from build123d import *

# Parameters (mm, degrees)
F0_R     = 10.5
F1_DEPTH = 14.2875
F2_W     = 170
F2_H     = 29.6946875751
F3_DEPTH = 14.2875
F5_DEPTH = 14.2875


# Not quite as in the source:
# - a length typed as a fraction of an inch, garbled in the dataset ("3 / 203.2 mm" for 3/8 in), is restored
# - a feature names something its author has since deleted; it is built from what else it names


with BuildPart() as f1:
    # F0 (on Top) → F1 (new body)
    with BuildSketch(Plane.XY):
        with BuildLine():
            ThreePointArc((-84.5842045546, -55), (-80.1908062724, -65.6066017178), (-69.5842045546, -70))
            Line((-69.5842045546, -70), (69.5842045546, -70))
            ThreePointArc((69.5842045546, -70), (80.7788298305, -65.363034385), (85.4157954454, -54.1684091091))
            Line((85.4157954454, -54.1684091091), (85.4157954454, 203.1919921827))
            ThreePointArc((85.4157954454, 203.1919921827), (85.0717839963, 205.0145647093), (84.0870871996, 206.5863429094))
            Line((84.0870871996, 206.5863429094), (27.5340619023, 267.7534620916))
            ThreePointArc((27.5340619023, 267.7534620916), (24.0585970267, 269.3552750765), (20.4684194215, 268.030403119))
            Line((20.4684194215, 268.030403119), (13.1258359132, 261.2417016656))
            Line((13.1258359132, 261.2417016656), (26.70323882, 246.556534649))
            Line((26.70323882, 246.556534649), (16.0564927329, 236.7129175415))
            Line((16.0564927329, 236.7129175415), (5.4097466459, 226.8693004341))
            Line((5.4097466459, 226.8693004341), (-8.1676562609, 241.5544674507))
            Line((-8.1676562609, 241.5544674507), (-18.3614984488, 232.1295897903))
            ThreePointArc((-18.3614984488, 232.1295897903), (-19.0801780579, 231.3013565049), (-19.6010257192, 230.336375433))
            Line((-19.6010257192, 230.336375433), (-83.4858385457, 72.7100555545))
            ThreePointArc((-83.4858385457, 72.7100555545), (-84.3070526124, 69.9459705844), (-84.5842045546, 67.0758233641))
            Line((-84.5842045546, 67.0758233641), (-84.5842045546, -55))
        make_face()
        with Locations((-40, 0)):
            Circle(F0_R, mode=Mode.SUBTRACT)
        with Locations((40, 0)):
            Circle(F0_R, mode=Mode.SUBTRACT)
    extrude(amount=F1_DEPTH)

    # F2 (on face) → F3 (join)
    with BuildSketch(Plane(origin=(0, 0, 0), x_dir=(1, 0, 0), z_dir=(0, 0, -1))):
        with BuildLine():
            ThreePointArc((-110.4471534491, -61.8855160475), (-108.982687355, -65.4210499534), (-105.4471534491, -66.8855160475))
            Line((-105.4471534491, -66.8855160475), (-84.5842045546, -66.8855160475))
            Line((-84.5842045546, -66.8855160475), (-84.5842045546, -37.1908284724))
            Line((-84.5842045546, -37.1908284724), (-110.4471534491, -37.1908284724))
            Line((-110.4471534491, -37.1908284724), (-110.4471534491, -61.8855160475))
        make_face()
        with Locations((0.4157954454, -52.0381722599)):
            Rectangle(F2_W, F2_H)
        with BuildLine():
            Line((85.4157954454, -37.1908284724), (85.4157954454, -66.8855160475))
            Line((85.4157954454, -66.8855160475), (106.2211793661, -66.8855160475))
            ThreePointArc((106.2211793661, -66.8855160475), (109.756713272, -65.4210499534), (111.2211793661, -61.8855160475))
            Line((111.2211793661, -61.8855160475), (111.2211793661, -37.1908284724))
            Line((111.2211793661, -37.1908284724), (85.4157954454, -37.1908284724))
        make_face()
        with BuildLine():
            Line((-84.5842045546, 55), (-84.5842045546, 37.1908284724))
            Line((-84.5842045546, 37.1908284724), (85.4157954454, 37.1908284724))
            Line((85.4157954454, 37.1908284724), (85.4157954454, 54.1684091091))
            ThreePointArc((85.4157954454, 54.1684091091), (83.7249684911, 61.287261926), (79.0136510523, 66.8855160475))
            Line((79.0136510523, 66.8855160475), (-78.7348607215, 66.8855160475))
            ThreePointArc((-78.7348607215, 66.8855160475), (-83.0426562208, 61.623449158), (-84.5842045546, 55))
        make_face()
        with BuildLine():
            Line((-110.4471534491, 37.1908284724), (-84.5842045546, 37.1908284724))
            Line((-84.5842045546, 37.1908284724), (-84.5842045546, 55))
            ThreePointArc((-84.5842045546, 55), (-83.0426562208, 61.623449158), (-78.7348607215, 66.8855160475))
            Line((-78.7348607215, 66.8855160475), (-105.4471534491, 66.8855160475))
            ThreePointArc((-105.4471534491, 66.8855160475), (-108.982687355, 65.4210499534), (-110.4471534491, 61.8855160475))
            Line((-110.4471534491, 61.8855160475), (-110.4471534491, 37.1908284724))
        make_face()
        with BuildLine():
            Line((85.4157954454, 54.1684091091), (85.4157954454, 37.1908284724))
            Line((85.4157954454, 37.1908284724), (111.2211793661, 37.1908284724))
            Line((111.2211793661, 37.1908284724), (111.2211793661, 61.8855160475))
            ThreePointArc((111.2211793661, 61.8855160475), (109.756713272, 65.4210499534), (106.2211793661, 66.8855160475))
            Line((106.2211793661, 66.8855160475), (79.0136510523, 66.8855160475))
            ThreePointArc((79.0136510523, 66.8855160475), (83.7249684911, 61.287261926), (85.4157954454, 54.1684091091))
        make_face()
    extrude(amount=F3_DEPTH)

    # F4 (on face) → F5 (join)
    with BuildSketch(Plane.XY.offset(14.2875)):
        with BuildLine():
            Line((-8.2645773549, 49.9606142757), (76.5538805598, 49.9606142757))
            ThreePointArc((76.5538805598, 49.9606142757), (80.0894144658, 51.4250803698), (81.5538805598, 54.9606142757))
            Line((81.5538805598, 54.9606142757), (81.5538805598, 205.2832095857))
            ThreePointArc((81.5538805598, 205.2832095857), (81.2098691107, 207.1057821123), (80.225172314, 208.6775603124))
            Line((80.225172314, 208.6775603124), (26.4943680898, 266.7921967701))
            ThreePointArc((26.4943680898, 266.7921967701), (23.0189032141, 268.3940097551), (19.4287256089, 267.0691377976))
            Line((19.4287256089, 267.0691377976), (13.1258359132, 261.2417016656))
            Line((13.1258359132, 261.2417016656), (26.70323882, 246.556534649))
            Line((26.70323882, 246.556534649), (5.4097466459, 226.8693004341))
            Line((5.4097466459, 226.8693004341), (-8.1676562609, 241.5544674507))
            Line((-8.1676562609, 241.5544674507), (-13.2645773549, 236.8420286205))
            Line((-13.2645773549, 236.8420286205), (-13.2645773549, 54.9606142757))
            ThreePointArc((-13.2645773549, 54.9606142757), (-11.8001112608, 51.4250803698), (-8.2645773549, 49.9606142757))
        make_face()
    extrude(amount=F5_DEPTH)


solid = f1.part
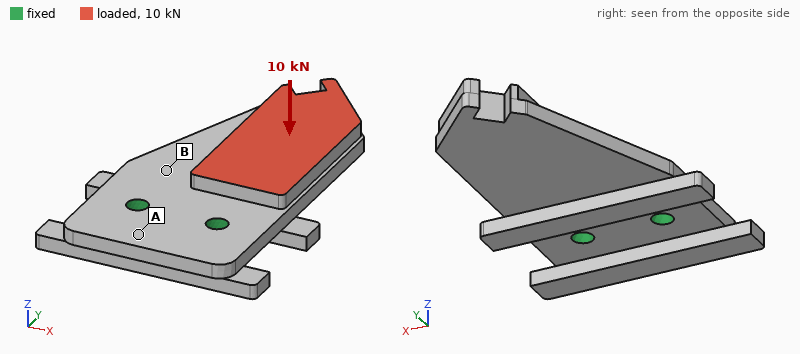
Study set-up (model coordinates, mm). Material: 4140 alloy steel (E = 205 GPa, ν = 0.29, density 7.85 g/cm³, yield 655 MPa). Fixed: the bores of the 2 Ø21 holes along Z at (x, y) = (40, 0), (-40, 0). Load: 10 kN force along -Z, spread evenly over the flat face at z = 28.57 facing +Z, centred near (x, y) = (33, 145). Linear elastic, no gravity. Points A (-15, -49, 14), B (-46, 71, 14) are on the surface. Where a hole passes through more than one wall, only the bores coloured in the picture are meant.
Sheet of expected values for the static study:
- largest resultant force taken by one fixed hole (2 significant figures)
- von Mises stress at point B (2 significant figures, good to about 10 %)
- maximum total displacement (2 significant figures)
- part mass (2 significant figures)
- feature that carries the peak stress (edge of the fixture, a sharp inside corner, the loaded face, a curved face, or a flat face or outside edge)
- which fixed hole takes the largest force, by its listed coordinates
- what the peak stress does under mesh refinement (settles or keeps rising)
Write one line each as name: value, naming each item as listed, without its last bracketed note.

largest resultant force taken by one fixed hole: 8.2 kN
von Mises stress at point B: 64 MPa
maximum total displacement: 1.7 mm
part mass: 8.6 kg
feature that carries the peak stress: edge of the fixture
which fixed hole takes the largest force, by its listed coordinates: (40, 0)
what the peak stress does under mesh refinement: keeps rising
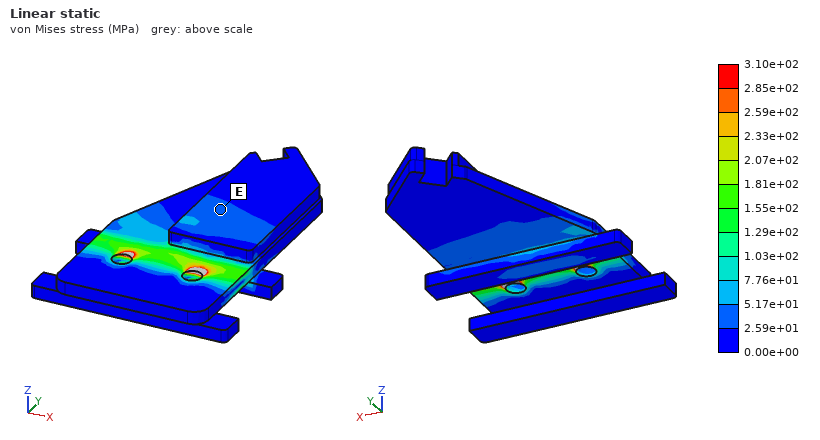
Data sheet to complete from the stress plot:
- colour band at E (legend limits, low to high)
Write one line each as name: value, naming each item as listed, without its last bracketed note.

colour band at E: 2.59e+01 to 5.17e+01 MPa
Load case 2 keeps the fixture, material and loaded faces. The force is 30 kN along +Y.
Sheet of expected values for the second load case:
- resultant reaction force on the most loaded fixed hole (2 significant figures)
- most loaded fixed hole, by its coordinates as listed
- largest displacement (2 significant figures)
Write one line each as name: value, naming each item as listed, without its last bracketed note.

resultant reaction force on the most loaded fixed hole: 26 kN
most loaded fixed hole, by its coordinates as listed: (40, 0)
largest displacement: 0.97 mm
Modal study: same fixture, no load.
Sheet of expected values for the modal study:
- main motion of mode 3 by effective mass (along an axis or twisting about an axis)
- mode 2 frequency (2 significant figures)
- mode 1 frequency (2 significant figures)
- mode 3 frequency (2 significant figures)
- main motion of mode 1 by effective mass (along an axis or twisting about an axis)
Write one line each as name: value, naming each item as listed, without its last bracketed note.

main motion of mode 3 by effective mass: along X
mode 2 frequency: 1300 Hz
mode 1 frequency: 230 Hz
mode 3 frequency: 1500 Hz
main motion of mode 1 by effective mass: along Z
